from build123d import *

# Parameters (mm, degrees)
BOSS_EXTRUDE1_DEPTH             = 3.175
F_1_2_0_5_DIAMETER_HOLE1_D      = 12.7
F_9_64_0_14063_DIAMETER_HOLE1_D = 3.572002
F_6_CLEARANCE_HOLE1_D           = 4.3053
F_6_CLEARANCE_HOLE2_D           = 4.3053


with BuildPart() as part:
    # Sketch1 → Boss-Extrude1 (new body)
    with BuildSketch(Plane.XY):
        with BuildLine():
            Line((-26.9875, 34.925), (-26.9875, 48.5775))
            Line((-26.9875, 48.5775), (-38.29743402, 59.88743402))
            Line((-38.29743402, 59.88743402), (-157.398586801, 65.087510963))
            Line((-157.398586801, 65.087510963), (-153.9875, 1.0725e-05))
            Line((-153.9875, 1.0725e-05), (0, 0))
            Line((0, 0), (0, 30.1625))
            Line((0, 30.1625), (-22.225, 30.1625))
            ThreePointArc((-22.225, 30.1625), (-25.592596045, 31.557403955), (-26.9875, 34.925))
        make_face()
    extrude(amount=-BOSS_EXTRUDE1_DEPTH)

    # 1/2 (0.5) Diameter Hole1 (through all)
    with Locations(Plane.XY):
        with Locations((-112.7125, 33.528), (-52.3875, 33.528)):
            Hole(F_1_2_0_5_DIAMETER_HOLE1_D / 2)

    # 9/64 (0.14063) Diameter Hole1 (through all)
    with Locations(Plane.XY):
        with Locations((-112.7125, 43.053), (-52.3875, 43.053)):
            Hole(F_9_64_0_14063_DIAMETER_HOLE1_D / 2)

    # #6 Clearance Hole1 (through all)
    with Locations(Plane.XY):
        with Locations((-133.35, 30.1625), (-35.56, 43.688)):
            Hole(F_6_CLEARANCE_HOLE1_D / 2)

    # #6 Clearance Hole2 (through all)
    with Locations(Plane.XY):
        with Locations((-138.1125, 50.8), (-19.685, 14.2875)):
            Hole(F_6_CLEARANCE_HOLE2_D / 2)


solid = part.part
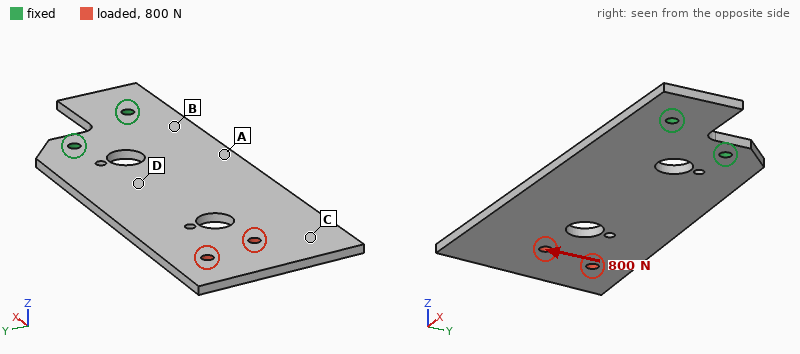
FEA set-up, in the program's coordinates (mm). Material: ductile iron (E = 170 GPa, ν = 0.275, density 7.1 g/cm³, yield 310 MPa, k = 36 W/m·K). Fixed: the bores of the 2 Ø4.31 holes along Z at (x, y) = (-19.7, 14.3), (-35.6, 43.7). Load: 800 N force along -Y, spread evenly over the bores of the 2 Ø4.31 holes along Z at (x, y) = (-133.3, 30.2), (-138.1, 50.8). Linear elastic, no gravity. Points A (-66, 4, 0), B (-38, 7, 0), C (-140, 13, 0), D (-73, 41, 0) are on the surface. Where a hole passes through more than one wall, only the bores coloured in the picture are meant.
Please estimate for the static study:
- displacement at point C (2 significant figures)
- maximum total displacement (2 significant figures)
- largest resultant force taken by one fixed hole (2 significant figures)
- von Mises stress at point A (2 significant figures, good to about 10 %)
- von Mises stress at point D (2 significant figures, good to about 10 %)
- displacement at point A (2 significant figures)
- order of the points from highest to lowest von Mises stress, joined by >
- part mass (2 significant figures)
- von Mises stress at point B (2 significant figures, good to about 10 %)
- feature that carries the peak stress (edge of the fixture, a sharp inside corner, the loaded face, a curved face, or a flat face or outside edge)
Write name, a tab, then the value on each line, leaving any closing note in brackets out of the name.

displacement at point C	68 µm
maximum total displacement	81 µm
largest resultant force taken by one fixed hole	2.6 kN
von Mises stress at point A	25 MPa
von Mises stress at point D	16 MPa
displacement at point A	21 µm
order of the points from highest to lowest von Mises stress, joined by >	B > A > D > C
part mass	190 g
von Mises stress at point B	35 MPa
feature that carries the peak stress	edge of the fixture
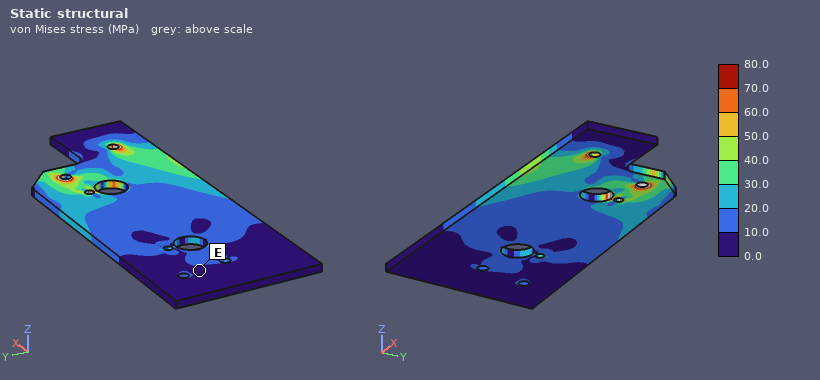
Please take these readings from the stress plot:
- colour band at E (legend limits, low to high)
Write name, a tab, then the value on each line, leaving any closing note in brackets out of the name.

colour band at E	0.0 to 10.0 MPa
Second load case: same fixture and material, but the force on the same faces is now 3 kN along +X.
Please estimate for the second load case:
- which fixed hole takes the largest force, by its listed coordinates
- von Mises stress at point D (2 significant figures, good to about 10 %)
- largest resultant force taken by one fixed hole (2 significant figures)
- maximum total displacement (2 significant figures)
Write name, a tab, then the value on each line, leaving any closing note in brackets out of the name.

which fixed hole takes the largest force, by its listed coordinates	(-35.6, 43.7)
von Mises stress at point D	19 MPa
largest resultant force taken by one fixed hole	2.5 kN
maximum total displacement	40 µm
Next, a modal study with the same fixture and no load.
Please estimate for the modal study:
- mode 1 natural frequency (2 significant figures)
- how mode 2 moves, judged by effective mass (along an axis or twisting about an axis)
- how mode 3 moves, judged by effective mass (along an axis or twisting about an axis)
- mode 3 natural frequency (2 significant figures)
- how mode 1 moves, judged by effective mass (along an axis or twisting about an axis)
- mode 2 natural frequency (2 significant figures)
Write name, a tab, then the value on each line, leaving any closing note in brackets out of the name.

mode 1 natural frequency	150 Hz
how mode 2 moves, judged by effective mass	twisting about X
how mode 3 moves, judged by effective mass	along Z
mode 3 natural frequency	970 Hz
how mode 1 moves, judged by effective mass	along Z
mode 2 natural frequency	610 Hz
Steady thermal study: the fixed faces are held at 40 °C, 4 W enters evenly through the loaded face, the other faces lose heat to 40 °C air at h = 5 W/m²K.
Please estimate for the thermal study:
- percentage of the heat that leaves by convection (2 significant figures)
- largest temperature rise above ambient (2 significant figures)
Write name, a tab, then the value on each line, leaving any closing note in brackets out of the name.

percentage of the heat that leaves by convection	50 %
largest temperature rise above ambient	48 K
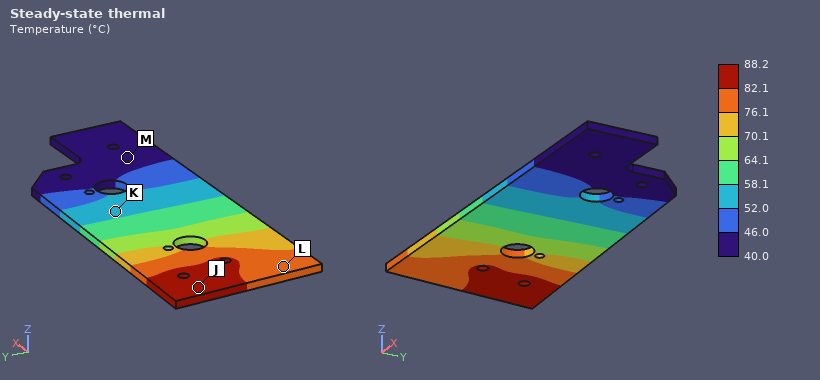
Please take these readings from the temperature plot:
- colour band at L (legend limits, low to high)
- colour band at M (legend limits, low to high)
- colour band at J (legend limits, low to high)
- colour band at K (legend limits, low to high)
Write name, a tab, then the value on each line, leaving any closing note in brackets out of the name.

colour band at L	76.1 to 82.1 °C
colour band at M	40.0 to 46.0 °C
colour band at J	82.1 to 88.2 °C
colour band at K	52.0 to 58.1 °C
